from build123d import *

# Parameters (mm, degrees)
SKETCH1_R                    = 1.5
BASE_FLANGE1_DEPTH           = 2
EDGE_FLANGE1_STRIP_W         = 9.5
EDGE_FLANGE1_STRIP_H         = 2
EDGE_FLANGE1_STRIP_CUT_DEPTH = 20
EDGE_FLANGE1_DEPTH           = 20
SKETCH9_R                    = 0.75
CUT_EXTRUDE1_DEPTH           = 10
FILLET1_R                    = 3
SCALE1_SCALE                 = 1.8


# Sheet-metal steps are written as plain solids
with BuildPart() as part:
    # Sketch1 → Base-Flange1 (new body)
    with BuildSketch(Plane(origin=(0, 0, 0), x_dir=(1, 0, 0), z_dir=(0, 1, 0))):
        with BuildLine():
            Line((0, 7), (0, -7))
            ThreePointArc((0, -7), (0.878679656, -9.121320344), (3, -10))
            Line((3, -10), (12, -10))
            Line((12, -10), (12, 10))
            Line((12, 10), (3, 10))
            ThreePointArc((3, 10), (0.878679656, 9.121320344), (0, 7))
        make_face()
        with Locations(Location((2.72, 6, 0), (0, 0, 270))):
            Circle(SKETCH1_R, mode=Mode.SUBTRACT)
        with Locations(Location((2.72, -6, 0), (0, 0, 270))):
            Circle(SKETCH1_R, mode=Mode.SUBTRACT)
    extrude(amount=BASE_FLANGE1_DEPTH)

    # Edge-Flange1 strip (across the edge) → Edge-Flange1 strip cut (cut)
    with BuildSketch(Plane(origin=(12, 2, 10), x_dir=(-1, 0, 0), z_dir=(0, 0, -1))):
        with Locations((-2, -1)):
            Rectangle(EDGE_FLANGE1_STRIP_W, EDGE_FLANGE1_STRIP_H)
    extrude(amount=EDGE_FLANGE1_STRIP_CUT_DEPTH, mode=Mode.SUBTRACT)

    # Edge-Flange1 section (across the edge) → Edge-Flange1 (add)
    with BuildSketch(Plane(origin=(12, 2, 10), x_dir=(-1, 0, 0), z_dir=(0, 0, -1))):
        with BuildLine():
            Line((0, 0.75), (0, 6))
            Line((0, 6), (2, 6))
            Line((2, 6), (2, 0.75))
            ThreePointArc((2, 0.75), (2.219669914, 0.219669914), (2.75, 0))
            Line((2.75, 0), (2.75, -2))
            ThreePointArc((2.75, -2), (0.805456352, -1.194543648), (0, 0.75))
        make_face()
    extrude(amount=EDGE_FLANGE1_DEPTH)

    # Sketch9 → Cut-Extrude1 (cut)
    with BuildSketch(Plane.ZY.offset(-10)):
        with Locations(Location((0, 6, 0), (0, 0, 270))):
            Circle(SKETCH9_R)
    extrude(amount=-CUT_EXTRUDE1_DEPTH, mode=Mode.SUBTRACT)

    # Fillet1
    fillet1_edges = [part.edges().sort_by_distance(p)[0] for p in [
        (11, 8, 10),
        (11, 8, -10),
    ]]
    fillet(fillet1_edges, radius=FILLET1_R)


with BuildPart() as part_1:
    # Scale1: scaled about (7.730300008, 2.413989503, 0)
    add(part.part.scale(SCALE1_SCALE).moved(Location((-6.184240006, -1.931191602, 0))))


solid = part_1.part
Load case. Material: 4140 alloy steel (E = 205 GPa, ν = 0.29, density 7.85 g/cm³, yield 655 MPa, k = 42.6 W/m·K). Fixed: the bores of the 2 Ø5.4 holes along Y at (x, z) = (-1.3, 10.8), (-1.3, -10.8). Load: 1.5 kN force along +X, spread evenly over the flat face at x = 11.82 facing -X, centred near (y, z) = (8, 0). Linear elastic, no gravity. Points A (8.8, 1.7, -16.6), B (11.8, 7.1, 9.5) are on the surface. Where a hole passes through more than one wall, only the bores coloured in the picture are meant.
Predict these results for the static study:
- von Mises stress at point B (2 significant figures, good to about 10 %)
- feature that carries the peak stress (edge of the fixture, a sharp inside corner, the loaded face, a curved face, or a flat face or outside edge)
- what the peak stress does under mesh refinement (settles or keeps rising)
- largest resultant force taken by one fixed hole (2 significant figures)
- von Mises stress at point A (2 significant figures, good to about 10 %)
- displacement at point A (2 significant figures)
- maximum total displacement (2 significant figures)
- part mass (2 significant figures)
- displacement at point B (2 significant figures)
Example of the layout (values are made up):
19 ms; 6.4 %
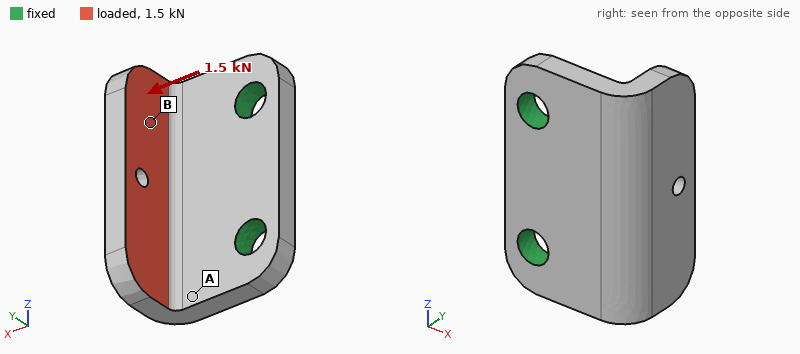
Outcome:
30 MPa; edge of the fixture; keeps rising; 760 N; 150 MPa; 17 µm; 92 µm; 29 g; 50 µm
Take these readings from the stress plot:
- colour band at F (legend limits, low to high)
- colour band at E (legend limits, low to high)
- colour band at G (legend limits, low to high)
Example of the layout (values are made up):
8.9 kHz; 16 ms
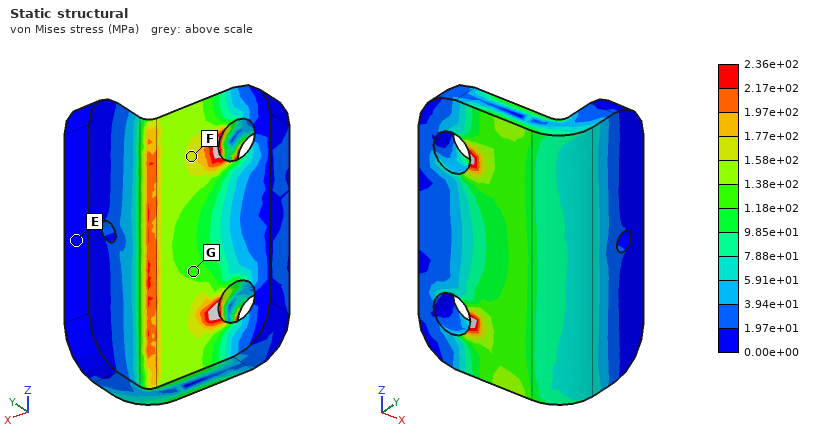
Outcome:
1.58e+02 to 1.77e+02 MPa; 0.00e+00 to 1.97e+01 MPa; 1.18e+02 to 1.38e+02 MPa
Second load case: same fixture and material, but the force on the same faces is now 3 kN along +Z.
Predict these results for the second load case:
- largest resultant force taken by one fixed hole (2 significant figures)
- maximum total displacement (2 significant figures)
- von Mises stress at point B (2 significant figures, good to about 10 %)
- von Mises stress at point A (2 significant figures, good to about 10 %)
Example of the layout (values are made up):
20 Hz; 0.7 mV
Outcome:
2.2 kN; 66 µm; 110 MPa; 110 MPa
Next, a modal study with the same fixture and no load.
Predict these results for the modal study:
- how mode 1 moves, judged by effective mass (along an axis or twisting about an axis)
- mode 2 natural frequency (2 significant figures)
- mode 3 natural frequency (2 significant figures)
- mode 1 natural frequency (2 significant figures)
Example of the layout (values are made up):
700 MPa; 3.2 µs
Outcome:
along Y; 9700 Hz; 17 kHz; 6000 Hz
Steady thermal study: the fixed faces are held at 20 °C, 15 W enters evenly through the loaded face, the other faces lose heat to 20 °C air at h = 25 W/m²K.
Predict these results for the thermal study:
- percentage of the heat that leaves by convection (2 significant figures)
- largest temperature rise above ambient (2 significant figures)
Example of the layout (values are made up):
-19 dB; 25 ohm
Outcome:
9.0 %; 55 K
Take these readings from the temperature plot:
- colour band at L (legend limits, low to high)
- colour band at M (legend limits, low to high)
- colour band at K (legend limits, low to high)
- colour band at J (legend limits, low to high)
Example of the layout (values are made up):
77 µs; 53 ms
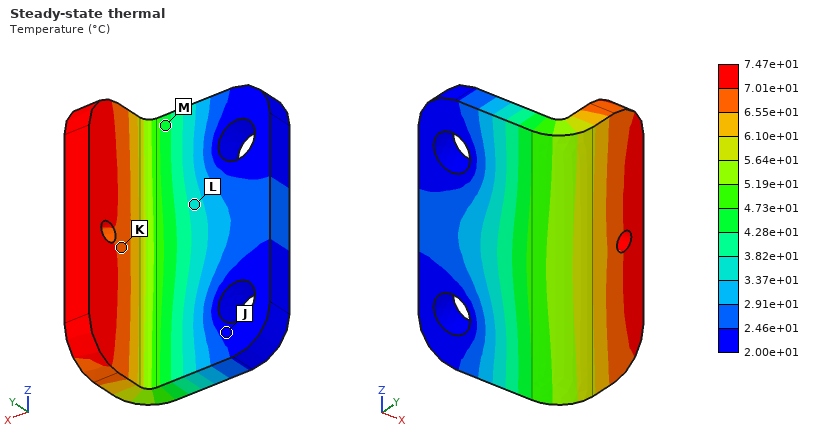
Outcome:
3.37e+01 to 3.82e+01 °C; 4.28e+01 to 4.73e+01 °C; 6.55e+01 to 7.01e+01 °C; 2.00e+01 to 2.46e+01 °C
